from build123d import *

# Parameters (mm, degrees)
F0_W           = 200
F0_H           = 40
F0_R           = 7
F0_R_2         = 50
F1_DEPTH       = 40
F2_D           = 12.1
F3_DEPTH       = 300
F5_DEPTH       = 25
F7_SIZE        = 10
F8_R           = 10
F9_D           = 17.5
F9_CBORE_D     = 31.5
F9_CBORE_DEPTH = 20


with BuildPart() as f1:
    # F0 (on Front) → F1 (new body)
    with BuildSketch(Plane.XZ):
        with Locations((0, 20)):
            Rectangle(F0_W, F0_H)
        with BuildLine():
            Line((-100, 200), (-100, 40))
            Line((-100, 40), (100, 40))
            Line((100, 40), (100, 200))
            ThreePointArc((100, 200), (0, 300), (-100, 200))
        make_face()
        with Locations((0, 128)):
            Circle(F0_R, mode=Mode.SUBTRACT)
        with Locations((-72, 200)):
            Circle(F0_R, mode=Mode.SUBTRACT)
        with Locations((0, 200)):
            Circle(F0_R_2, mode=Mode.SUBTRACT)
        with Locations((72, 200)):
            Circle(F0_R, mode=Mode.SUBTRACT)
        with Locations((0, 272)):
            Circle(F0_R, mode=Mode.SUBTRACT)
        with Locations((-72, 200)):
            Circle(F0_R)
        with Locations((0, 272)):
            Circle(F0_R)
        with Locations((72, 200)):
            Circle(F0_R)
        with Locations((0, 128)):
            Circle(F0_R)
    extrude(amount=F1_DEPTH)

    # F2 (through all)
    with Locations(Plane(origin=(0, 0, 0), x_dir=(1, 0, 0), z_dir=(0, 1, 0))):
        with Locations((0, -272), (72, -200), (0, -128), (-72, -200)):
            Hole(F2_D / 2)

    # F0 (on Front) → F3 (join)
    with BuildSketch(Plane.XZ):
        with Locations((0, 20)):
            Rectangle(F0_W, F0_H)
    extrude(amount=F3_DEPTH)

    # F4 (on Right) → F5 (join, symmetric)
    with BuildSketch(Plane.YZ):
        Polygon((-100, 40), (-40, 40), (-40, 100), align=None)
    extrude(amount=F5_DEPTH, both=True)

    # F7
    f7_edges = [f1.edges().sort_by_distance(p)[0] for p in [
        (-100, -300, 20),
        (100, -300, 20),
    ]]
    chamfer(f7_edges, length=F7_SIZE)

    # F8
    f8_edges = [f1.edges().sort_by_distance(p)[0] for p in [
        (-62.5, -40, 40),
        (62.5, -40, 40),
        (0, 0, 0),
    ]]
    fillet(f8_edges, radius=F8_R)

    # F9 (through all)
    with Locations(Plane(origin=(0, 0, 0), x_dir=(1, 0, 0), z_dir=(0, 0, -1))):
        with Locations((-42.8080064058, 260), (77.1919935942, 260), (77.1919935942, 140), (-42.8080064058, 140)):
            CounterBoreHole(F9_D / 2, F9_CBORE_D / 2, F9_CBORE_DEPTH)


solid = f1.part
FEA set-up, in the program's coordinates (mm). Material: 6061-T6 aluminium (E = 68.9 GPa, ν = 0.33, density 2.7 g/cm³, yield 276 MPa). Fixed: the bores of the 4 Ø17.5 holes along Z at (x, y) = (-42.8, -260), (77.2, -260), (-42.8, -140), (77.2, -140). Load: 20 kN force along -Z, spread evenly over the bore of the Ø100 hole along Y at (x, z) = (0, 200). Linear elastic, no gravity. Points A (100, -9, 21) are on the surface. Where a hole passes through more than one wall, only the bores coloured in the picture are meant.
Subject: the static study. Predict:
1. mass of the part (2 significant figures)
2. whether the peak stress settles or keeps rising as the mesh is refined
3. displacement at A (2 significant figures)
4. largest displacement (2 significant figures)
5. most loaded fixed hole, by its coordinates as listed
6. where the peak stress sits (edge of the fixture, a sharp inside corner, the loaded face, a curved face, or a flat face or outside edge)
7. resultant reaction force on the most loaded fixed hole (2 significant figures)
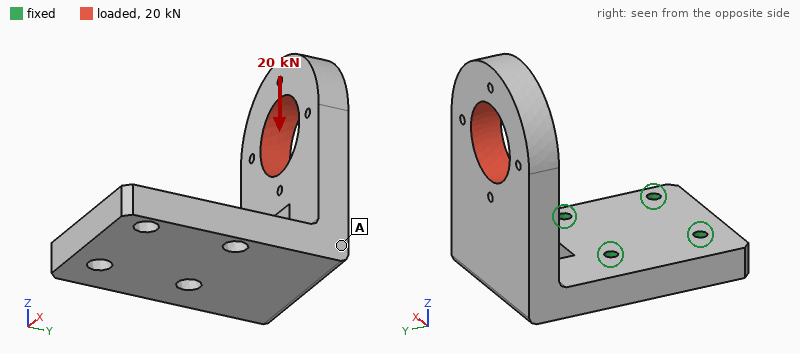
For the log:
11 kg
keeps rising
0.30 mm
0.80 mm
(-42.8, -140)
edge of the fixture
25 kN
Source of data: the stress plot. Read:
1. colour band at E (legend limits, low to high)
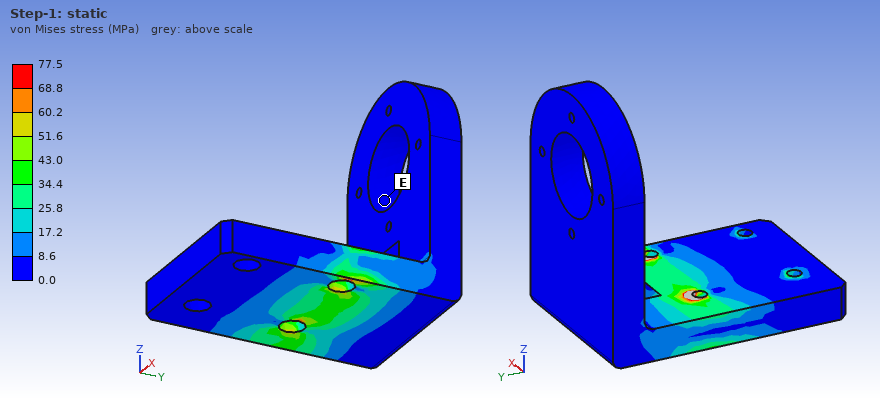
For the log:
0.0 to 8.6 MPa
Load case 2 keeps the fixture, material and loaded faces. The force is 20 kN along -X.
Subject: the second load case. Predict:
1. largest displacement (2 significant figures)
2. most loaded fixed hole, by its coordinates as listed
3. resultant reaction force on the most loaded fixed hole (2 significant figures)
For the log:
0.74 mm
(-42.8, -140)
36 kN
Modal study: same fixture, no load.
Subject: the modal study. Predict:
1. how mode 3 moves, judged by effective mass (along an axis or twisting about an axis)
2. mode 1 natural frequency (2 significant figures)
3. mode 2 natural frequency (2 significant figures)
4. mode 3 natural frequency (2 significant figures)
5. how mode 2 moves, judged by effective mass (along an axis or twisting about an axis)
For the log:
along Z
320 Hz
550 Hz
960 Hz
along X
